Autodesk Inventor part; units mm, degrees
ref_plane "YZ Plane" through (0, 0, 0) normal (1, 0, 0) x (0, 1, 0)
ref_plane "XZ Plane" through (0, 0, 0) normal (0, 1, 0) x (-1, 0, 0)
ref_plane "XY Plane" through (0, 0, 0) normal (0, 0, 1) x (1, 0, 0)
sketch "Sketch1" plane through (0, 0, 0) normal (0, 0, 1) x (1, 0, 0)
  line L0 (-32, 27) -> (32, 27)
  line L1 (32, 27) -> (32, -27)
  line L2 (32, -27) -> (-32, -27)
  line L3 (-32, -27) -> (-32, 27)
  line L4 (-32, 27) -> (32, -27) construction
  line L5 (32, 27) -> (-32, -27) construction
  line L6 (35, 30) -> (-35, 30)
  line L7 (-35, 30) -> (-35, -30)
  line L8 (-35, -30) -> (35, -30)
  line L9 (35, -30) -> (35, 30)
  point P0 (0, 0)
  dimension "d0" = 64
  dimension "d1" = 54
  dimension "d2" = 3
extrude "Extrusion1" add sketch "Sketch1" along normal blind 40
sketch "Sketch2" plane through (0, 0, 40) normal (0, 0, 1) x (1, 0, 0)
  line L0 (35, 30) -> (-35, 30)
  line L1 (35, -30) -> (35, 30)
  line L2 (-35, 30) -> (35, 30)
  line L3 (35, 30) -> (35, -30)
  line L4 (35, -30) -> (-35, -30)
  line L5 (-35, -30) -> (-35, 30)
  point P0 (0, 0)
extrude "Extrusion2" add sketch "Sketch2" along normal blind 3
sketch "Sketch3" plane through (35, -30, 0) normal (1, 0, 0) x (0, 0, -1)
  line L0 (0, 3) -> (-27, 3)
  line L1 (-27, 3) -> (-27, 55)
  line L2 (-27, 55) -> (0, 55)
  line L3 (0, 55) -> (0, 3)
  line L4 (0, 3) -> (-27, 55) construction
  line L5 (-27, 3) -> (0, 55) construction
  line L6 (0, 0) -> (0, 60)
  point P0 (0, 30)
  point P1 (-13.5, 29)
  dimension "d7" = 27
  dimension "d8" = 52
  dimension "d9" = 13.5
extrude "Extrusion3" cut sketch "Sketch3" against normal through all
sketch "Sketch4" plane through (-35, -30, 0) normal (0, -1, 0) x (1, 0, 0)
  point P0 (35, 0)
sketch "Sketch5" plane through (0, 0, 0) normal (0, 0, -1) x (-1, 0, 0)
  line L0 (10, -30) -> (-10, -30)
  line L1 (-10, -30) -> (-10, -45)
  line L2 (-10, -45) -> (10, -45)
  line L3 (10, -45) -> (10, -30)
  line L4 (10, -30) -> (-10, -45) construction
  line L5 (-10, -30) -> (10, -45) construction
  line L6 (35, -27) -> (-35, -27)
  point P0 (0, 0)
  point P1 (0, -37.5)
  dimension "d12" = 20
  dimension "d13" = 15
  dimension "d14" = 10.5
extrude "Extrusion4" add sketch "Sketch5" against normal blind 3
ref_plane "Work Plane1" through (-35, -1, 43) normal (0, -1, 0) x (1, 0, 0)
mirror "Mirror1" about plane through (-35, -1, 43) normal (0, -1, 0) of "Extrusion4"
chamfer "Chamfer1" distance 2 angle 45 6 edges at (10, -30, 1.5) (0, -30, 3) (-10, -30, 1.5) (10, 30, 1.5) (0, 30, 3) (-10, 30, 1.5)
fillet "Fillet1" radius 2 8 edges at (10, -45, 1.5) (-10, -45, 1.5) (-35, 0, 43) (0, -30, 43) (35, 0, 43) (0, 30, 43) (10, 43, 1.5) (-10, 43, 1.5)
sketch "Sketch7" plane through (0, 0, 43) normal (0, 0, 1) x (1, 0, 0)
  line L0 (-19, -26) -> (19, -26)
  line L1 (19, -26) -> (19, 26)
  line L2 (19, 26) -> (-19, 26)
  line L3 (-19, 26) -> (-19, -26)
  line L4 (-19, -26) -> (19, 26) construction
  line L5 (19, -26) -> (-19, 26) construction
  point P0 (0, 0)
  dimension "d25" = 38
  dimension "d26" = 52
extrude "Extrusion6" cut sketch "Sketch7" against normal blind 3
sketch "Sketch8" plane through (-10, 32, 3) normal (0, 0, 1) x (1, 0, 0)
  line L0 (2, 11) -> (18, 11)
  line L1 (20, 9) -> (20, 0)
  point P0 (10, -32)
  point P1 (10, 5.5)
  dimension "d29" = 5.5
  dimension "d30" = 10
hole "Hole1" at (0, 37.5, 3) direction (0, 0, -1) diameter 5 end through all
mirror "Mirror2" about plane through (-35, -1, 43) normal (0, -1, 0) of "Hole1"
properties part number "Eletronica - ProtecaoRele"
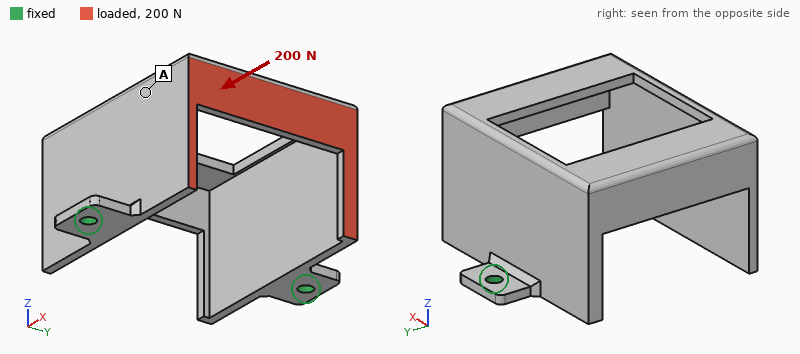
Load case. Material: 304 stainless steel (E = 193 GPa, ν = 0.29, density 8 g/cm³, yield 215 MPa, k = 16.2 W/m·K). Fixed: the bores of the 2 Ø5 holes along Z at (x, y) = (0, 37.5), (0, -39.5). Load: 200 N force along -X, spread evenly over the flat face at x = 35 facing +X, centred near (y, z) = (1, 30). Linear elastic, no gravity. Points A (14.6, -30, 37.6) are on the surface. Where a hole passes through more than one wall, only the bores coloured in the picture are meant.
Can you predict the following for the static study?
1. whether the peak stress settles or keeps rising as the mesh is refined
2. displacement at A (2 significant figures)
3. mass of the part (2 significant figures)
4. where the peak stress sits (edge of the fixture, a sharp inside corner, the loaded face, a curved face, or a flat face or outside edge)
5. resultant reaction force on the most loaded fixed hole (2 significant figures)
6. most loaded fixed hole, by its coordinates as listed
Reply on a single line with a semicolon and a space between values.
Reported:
keeps rising; 47 µm; 240 g; edge of the fixture; 110 N; (0, 37.5)
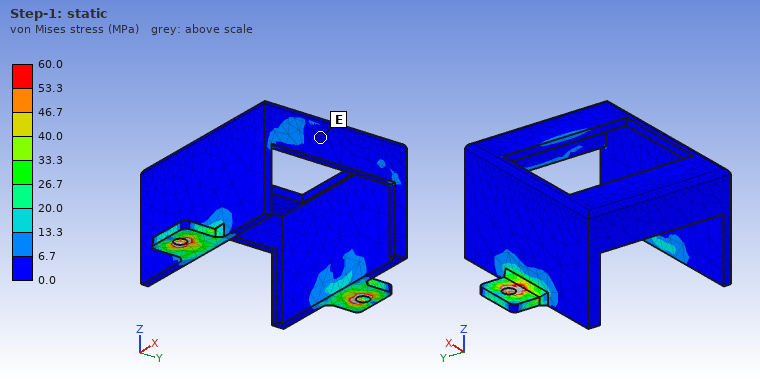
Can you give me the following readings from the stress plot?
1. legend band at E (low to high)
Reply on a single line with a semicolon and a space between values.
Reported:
0.0 to 6.7 MPa
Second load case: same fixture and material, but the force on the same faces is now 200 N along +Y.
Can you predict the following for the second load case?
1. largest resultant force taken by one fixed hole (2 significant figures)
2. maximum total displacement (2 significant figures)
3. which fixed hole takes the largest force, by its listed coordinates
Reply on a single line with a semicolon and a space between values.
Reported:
140 N; 60 µm; (0, 37.5)
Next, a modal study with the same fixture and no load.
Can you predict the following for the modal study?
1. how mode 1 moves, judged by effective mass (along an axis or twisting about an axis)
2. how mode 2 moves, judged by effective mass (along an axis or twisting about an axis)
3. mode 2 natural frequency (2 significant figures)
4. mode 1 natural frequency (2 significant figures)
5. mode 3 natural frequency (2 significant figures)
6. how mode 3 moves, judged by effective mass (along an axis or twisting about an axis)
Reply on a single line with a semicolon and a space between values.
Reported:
along X; along Y; 1100 Hz; 630 Hz; 1200 Hz; twisting about Z
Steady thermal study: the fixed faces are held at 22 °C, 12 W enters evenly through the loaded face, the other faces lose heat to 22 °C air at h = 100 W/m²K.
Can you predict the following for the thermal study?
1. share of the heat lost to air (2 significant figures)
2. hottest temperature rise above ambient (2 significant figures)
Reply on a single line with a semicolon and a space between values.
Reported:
98 %; 39 K
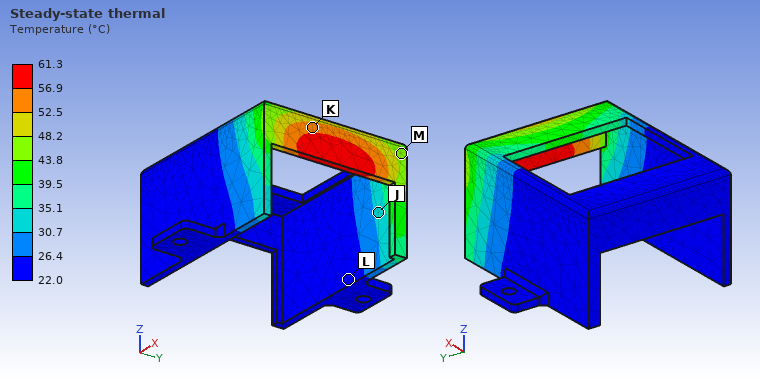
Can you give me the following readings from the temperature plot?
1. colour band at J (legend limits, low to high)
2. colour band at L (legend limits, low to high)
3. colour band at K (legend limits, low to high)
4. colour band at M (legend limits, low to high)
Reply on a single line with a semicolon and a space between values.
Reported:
30.7 to 35.1 °C; 22.0 to 26.4 °C; 52.5 to 56.9 °C; 43.8 to 48.2 °C
